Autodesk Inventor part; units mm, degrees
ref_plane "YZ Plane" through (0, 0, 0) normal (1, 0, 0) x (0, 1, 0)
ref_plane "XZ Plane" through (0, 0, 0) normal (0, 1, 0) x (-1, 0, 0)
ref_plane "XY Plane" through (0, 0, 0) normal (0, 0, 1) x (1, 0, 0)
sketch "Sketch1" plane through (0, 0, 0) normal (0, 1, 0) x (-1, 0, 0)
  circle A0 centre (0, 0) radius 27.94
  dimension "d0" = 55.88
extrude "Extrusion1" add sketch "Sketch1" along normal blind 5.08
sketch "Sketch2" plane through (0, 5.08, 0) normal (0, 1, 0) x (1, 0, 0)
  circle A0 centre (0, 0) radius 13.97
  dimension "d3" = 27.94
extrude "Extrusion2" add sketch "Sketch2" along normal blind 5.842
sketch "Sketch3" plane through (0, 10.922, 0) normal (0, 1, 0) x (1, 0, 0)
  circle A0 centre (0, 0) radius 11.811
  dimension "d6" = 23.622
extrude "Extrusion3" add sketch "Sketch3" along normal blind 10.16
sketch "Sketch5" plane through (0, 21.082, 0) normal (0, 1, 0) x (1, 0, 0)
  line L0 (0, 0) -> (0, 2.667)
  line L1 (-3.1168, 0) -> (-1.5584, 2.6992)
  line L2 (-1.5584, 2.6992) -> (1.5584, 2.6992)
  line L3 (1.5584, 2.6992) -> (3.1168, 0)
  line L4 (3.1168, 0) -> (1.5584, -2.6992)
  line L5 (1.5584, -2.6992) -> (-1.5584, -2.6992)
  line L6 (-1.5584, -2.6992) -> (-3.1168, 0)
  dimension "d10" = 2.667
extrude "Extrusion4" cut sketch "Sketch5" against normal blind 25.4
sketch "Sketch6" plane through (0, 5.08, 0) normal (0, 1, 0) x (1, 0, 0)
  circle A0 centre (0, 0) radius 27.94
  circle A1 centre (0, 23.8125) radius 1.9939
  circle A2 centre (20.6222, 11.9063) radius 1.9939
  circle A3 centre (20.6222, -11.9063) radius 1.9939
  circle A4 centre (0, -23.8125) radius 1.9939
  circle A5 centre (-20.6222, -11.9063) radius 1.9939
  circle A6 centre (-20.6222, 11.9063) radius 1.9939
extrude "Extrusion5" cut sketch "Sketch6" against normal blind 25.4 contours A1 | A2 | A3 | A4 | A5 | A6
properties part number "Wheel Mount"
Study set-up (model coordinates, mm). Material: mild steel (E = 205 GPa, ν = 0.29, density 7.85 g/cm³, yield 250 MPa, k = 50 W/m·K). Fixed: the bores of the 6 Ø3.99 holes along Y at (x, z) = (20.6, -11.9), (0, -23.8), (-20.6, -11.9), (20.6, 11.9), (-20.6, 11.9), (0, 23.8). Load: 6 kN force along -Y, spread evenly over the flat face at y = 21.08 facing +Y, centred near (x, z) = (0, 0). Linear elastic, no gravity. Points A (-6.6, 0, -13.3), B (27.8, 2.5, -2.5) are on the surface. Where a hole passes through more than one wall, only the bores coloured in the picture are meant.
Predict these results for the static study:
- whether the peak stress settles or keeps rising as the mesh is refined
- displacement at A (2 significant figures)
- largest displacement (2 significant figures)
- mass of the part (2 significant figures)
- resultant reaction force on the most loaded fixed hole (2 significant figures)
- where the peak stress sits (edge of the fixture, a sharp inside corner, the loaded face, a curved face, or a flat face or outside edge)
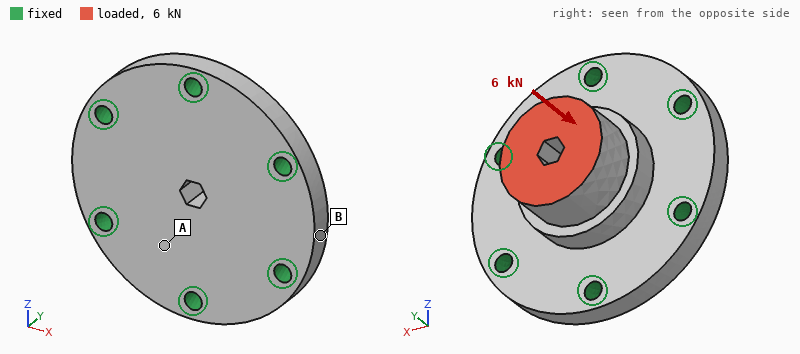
keeps rising
5.4 µm
7.7 µm
150 g
1.1 kN
edge of the fixture
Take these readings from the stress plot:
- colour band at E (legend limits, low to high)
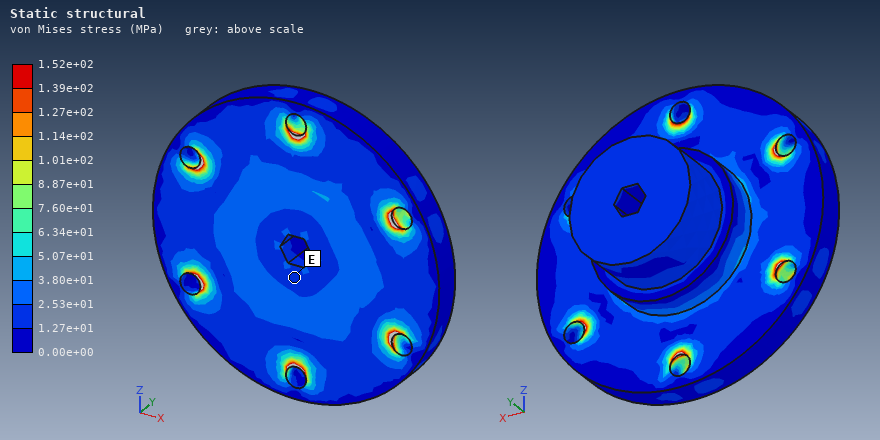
1.27e+01 to 2.53e+01 MPa
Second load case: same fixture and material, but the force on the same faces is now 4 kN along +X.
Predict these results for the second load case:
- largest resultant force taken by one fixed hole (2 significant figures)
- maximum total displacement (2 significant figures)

1.4 kN
13 µm
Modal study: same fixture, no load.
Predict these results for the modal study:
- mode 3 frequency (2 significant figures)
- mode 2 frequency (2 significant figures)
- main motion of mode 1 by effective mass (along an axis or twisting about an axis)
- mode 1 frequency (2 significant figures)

18 kHz
18 kHz
along Y
15 kHz
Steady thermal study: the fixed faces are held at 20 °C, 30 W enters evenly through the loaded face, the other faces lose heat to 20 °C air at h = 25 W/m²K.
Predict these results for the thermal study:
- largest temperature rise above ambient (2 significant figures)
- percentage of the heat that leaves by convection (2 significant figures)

37 K
6.1 %
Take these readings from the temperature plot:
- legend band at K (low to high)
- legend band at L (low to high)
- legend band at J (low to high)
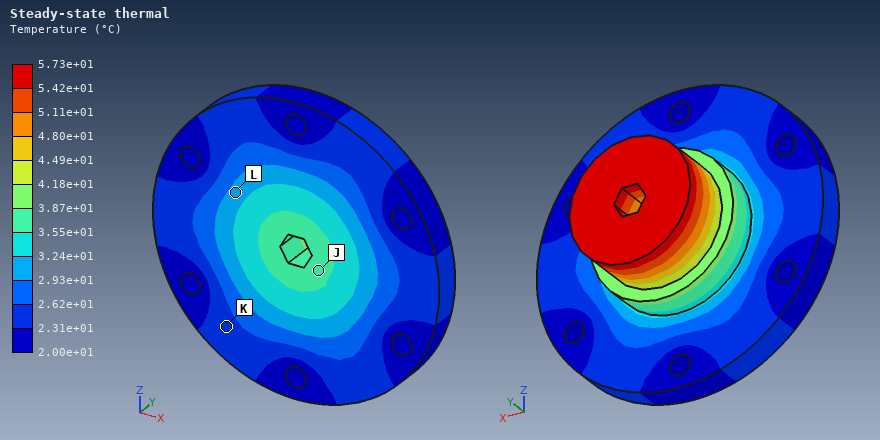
2.31e+01 to 2.62e+01 °C
2.93e+01 to 3.24e+01 °C
3.55e+01 to 3.87e+01 °C
